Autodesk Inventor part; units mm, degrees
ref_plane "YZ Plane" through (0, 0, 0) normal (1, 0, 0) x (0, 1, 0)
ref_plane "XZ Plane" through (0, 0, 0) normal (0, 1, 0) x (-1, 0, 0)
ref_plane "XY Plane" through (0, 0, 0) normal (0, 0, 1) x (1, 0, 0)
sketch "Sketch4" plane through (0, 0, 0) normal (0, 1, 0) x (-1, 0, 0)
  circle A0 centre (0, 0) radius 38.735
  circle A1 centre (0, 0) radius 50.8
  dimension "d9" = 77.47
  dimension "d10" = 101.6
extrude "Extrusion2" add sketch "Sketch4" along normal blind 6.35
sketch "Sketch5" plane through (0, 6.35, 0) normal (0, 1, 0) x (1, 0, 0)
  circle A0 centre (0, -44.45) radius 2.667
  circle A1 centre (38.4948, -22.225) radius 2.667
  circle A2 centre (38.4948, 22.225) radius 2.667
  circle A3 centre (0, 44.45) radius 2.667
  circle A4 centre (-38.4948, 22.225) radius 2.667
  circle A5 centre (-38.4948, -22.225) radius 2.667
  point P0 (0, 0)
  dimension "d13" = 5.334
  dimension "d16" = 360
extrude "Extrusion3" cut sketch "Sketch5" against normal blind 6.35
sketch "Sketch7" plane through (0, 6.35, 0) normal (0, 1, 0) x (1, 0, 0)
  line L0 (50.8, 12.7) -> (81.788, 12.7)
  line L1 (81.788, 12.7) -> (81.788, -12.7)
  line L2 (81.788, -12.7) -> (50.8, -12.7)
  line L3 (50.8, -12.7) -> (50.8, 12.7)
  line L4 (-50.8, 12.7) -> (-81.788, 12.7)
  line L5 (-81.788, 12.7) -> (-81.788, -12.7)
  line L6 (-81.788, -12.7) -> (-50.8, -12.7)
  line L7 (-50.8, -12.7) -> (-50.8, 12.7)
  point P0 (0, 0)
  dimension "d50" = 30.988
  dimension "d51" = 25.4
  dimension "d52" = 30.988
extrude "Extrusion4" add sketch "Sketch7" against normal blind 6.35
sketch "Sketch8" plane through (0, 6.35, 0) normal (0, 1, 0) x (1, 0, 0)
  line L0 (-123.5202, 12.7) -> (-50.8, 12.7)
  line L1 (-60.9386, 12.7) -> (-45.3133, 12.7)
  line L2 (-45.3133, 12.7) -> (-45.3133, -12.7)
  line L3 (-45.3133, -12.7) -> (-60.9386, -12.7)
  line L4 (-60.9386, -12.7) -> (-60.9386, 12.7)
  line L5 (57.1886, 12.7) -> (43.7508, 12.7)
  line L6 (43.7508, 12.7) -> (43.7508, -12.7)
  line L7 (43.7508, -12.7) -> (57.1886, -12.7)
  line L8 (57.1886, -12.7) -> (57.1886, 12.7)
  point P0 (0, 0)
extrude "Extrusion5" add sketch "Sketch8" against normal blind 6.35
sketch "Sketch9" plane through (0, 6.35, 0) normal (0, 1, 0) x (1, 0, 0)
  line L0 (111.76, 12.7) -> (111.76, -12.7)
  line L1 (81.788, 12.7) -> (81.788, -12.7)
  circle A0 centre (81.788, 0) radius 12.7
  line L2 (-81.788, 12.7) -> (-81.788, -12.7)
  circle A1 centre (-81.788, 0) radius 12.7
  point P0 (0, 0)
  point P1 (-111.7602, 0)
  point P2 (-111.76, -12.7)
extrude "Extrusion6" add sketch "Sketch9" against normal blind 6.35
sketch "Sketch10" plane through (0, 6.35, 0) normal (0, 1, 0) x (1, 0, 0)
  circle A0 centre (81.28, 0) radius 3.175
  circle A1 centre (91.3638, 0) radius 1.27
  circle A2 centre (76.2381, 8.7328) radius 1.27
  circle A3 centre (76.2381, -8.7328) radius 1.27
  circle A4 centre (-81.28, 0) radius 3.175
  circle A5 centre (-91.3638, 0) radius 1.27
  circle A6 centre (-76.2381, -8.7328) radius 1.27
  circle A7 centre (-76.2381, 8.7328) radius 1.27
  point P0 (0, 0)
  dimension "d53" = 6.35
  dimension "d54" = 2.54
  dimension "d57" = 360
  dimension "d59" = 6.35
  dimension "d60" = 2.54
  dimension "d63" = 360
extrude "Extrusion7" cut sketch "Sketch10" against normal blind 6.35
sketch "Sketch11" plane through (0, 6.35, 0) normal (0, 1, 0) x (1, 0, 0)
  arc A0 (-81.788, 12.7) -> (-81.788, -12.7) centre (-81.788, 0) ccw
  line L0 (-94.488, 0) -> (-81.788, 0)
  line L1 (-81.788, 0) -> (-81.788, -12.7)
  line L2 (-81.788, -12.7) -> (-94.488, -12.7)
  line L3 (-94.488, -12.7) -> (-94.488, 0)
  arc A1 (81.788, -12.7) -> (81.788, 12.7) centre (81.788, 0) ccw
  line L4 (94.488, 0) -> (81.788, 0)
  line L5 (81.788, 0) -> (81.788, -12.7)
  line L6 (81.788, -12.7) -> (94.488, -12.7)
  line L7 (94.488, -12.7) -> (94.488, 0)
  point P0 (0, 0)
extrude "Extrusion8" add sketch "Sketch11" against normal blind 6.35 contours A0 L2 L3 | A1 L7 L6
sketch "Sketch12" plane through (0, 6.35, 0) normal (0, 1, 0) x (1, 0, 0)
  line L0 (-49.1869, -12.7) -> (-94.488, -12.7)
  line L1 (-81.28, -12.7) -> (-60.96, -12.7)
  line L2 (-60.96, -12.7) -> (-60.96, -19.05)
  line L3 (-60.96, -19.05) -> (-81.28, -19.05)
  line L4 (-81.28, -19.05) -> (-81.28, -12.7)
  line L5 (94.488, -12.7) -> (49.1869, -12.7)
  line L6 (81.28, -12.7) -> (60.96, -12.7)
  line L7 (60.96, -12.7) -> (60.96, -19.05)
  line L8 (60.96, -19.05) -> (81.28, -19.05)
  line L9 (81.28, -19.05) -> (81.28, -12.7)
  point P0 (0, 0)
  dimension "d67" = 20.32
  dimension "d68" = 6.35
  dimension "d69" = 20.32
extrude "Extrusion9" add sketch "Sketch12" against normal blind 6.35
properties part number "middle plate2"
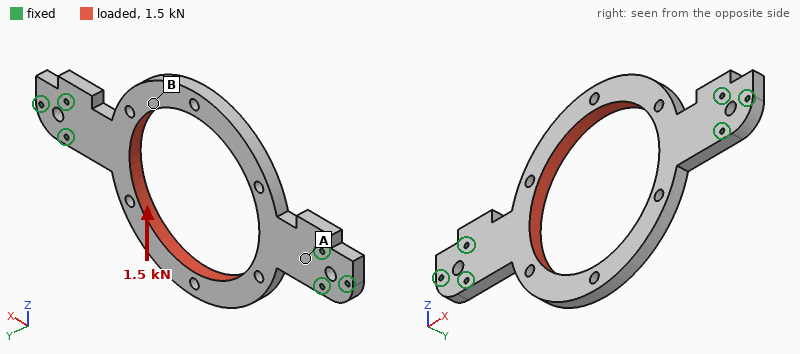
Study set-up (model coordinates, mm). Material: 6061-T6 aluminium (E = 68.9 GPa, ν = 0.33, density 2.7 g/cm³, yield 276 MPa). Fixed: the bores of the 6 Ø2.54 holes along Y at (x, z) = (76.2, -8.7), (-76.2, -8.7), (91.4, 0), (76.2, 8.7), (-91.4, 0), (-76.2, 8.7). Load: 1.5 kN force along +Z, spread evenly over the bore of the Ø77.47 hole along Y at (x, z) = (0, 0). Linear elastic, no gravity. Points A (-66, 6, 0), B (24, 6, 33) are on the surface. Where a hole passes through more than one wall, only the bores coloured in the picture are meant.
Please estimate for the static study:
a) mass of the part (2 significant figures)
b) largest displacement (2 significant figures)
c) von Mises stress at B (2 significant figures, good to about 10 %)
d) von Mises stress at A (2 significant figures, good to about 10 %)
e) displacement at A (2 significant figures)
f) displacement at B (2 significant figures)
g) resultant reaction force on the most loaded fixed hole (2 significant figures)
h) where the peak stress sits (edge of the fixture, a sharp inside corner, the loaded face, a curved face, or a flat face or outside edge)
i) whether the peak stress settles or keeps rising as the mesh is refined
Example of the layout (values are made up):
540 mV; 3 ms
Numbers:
96 g; 16 µm; 4.5 MPa; 11 MPa; 3.1 µm; 15 µm; 900 N; edge of the fixture; keeps rising
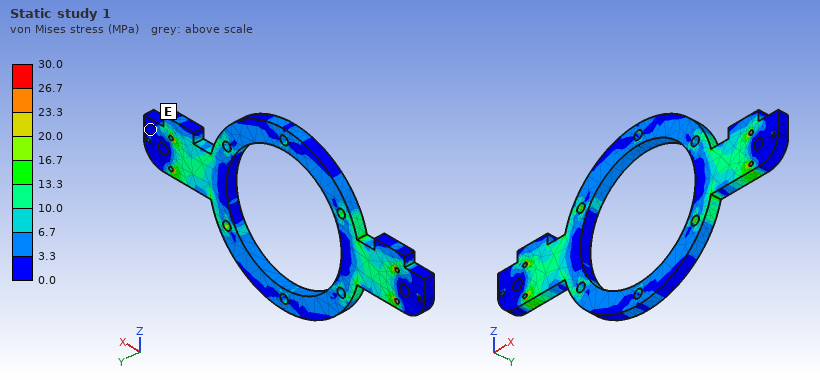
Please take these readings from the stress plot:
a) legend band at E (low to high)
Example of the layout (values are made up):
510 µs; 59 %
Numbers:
0.0 to 3.3 MPa
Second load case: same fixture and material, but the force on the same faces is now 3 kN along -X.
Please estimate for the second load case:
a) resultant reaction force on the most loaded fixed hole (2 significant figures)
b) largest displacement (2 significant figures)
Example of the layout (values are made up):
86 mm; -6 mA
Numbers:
720 N; 36 µm
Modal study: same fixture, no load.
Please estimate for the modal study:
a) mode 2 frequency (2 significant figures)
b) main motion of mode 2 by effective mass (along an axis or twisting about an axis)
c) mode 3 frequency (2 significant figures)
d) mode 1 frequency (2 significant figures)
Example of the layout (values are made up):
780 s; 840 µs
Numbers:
1100 Hz; along Y; 2700 Hz; 1000 Hz
